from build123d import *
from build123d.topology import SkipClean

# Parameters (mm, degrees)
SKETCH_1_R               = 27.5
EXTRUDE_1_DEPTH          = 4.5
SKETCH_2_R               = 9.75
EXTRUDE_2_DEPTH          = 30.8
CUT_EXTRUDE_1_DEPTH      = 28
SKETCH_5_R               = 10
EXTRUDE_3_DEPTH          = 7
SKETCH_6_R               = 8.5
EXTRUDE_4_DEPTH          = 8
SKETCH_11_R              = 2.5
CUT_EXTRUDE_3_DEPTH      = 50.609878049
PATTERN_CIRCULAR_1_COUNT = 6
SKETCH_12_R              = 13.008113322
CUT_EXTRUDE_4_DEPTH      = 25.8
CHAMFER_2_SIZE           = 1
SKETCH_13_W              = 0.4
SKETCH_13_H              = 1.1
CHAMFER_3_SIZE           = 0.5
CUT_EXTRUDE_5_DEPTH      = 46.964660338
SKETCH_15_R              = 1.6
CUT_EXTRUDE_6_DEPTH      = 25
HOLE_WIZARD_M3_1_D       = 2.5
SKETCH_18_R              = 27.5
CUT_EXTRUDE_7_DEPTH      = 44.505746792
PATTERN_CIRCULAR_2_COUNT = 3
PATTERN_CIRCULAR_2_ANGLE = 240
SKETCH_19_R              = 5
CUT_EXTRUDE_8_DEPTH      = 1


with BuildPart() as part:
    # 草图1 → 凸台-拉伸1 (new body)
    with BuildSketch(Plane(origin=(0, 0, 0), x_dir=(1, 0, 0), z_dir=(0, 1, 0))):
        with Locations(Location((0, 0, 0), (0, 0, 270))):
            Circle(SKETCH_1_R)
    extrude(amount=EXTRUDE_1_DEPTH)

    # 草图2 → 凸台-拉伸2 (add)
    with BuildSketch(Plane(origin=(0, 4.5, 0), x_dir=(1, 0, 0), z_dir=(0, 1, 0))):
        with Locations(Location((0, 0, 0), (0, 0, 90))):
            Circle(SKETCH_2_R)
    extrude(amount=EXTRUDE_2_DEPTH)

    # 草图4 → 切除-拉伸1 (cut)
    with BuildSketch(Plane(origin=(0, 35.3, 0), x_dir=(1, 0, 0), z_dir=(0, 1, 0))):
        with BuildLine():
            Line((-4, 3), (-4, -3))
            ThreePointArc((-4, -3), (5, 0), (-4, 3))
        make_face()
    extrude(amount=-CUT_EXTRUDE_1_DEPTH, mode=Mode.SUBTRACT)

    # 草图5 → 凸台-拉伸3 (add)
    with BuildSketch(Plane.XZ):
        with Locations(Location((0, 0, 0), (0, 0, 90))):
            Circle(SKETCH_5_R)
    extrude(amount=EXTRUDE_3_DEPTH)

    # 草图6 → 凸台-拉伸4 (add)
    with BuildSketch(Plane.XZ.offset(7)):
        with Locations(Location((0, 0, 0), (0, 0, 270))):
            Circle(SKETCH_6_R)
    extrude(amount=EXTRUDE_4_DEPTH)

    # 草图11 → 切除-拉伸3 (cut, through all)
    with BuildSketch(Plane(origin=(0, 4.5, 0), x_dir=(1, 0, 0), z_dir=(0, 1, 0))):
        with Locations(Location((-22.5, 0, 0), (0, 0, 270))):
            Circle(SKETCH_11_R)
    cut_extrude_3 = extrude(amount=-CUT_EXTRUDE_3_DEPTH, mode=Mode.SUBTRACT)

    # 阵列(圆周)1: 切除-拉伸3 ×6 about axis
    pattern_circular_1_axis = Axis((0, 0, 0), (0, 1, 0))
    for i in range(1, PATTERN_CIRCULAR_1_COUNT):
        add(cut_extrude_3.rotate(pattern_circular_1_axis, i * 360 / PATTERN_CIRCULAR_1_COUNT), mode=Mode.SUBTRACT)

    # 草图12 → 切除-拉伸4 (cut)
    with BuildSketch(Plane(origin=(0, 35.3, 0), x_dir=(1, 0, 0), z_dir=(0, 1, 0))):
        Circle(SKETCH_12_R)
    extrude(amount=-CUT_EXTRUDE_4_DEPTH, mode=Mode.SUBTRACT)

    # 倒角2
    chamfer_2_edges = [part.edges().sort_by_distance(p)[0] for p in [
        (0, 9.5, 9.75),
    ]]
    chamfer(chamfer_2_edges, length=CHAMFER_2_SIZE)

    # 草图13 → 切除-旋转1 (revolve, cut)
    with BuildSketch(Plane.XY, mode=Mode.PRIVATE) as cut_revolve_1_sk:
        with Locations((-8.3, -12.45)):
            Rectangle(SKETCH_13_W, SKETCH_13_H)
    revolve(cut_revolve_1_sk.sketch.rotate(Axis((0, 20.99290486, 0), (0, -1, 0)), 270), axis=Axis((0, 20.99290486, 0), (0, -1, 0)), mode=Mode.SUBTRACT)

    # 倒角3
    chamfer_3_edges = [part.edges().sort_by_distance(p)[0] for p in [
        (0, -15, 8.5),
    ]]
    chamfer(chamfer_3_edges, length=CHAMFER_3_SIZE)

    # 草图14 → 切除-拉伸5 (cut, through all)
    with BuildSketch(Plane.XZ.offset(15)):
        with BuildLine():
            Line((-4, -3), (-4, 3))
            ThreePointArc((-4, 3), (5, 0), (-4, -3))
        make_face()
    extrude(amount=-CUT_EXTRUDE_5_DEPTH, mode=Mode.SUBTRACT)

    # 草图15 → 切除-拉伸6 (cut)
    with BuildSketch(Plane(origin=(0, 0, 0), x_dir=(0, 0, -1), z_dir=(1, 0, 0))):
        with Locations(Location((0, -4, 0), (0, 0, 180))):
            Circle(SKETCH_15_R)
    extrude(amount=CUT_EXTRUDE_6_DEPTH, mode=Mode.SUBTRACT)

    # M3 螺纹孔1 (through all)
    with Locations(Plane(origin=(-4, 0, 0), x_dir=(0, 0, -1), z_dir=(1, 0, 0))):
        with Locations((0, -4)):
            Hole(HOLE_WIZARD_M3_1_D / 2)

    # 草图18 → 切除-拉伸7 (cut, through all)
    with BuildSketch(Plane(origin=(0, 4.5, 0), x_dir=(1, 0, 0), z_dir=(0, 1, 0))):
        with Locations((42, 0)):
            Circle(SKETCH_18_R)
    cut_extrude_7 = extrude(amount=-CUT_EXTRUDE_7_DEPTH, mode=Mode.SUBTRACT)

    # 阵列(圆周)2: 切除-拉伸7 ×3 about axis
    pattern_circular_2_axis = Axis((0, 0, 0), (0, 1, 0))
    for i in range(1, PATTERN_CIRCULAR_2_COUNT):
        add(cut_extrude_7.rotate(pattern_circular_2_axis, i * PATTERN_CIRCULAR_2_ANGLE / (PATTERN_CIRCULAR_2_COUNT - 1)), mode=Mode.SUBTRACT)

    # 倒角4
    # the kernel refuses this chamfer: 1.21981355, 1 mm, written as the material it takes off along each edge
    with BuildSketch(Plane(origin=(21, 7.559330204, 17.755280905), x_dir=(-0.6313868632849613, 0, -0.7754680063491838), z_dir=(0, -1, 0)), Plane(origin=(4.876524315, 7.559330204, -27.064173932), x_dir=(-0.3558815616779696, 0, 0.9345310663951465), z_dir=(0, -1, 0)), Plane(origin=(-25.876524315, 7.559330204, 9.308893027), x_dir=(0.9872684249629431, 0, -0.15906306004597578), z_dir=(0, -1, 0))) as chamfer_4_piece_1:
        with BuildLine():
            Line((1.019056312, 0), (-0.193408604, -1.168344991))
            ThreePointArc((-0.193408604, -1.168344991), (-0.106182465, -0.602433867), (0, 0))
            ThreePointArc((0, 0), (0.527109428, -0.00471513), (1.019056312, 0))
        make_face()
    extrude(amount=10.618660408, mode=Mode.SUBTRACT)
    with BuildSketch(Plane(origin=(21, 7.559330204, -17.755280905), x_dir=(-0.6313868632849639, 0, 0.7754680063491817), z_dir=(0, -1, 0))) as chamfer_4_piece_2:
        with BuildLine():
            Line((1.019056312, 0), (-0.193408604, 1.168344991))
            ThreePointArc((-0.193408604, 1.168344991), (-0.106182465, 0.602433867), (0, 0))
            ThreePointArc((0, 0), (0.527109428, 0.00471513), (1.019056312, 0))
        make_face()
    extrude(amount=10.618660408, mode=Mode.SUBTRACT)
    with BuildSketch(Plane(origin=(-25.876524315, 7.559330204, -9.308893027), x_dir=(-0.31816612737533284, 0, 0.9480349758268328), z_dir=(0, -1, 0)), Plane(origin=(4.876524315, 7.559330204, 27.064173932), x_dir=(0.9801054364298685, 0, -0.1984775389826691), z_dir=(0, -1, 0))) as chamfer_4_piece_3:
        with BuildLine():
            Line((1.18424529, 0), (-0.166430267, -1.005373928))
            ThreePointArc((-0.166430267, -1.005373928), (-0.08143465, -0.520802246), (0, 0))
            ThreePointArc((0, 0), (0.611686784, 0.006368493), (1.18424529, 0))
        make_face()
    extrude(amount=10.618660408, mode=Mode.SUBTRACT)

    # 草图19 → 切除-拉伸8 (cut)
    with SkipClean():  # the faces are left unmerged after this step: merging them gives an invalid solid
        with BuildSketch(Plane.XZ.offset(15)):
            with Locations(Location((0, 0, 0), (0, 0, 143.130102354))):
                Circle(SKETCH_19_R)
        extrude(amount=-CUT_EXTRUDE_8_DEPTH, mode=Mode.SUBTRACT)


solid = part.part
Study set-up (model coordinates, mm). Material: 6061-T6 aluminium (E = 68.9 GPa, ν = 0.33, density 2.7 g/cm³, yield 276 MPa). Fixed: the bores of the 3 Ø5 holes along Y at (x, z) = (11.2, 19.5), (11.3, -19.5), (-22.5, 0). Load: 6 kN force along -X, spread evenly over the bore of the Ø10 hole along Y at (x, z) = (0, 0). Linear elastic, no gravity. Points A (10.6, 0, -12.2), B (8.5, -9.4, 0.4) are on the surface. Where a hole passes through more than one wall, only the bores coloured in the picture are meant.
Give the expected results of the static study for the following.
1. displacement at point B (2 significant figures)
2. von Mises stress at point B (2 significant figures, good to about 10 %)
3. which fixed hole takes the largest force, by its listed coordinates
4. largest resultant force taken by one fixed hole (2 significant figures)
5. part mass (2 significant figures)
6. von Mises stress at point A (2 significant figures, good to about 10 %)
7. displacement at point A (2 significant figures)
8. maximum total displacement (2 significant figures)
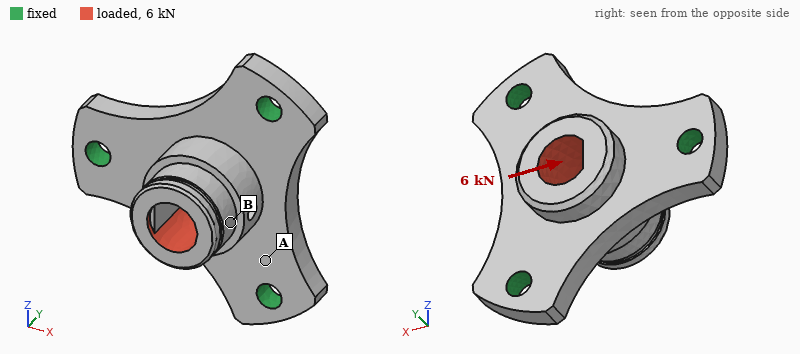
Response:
54 µm
24 MPa
(-22.5, 0)
3.2 kN
26 g
49 MPa
12 µm
69 µm
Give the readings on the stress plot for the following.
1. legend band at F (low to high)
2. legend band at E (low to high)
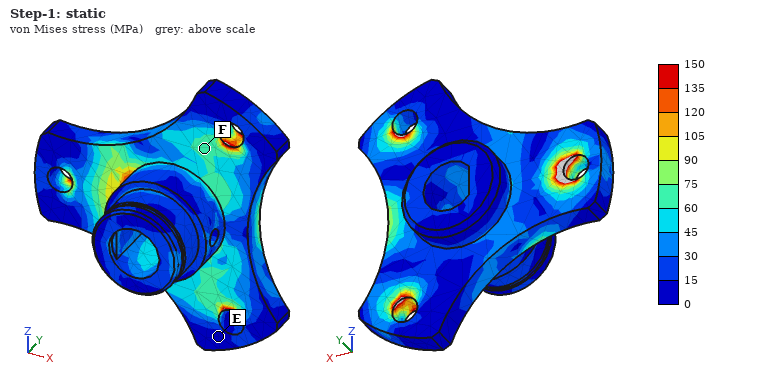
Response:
60 to 75 MPa
0 to 15 MPa
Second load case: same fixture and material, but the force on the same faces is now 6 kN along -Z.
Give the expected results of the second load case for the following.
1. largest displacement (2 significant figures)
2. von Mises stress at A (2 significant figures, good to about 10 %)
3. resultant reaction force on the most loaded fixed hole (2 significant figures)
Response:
66 µm
67 MPa
2.9 kN
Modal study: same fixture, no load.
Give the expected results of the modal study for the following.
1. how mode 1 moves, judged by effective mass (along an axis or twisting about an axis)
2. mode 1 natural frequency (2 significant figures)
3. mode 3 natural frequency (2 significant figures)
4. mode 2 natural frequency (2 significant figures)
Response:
along Y
12 kHz
14 kHz
14 kHz
